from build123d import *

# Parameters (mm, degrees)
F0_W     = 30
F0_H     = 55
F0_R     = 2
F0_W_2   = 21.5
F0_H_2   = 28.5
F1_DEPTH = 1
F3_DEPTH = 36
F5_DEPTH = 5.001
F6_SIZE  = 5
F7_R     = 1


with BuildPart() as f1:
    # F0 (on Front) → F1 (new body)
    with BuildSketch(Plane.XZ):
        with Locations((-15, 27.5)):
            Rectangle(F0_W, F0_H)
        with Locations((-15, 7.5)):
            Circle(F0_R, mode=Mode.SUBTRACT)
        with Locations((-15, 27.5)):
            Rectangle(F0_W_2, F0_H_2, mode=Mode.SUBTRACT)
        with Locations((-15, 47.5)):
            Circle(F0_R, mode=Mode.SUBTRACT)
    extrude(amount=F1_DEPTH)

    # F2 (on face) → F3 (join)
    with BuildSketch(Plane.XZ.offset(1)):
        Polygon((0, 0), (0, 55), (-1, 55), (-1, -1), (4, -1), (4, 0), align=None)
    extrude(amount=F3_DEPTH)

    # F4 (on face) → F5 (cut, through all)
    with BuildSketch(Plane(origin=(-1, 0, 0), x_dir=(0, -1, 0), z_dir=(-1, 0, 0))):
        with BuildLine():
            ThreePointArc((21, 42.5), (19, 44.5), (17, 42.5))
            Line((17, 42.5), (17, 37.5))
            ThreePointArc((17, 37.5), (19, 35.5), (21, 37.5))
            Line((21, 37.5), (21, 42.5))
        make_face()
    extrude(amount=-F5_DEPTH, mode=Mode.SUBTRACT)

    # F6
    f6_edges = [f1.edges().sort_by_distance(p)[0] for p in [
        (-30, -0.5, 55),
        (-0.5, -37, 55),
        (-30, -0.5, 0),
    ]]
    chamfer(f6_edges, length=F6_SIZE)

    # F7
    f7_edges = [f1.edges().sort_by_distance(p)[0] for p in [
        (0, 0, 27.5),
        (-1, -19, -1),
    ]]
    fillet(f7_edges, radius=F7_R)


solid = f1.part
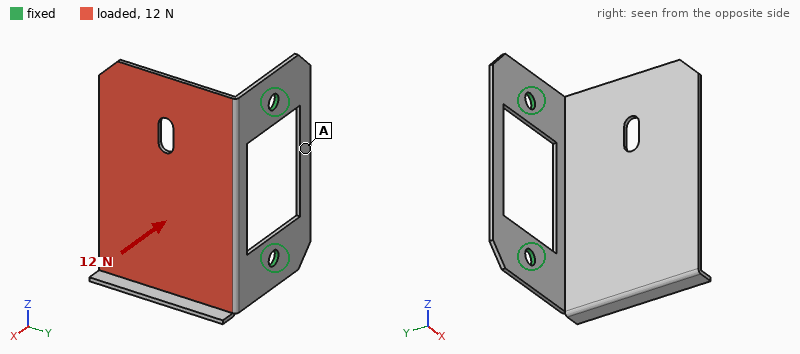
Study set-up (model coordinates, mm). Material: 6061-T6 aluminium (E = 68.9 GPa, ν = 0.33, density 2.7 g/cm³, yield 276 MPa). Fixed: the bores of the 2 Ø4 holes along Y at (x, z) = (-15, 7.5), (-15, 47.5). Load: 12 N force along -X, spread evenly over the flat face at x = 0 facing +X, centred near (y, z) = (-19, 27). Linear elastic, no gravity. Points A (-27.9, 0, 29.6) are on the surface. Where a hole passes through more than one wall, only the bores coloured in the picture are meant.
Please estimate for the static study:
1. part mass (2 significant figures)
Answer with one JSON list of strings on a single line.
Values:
["8.3 g"]
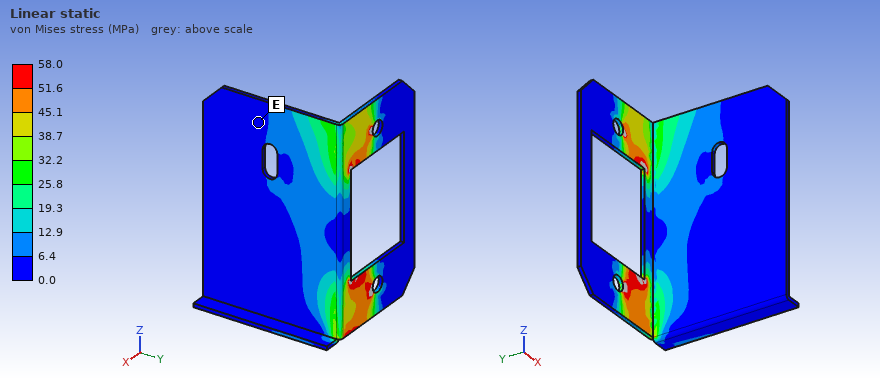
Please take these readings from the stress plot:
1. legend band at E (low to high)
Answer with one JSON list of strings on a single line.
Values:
["0.0 to 6.4 MPa"]
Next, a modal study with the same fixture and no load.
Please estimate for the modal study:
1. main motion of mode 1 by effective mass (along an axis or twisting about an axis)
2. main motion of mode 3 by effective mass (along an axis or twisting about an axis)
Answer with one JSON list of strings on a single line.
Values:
["along X", "along Z"]
